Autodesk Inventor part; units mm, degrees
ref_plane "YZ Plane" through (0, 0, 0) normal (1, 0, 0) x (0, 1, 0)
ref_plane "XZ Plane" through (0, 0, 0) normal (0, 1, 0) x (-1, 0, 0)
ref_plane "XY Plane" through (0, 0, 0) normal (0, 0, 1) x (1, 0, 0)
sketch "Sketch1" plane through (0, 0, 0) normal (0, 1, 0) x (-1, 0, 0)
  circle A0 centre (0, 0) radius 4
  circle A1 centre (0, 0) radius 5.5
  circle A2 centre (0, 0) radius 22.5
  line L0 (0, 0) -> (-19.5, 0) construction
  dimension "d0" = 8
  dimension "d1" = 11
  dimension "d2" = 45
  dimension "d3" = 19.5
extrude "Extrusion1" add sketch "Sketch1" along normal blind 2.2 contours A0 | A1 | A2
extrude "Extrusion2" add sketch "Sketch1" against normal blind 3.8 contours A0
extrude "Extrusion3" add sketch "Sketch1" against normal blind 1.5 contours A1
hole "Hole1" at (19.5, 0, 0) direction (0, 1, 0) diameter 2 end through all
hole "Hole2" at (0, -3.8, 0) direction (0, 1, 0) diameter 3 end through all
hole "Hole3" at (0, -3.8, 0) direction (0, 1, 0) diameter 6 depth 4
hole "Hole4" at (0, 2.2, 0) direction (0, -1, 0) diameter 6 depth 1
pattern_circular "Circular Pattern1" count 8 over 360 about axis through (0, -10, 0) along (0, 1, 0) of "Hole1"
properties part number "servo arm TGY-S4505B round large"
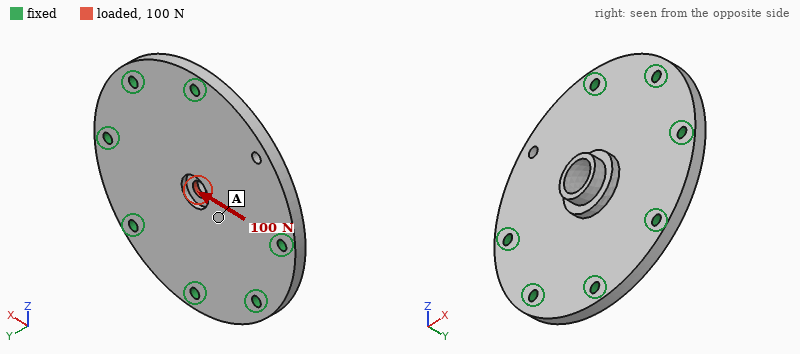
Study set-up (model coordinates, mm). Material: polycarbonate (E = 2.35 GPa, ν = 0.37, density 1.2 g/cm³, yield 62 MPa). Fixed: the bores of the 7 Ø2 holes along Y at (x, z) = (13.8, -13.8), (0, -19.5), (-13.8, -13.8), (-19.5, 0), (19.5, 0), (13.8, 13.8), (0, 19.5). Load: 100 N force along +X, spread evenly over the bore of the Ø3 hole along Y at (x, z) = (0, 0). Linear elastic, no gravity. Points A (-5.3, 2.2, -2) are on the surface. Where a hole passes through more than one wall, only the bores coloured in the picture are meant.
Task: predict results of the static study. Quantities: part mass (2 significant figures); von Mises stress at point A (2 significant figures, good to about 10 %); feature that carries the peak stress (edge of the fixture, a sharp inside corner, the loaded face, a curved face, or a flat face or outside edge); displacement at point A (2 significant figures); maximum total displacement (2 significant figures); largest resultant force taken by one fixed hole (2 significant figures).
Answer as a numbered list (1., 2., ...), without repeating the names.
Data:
1. 4.3 g
2. 1.6 MPa
3. the loaded face
4. 9.4 µm
5. 20 µm
6. 24 N
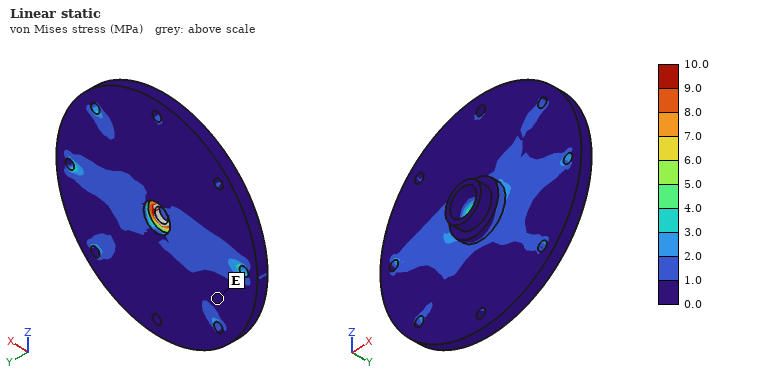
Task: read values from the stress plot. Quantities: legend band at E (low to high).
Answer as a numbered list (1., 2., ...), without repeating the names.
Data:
1. 0.0 to 1.0 MPa
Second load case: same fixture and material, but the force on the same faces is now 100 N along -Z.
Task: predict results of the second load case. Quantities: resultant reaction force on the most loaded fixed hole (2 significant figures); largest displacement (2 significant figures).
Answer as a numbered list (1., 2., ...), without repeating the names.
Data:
1. 24 N
2. 20 µm
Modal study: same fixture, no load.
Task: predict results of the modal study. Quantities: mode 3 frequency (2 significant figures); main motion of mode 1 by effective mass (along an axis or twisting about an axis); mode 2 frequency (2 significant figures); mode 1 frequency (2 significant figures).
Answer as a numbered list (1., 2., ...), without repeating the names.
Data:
1. 6700 Hz
2. along Y
3. 3700 Hz
4. 3200 Hz
